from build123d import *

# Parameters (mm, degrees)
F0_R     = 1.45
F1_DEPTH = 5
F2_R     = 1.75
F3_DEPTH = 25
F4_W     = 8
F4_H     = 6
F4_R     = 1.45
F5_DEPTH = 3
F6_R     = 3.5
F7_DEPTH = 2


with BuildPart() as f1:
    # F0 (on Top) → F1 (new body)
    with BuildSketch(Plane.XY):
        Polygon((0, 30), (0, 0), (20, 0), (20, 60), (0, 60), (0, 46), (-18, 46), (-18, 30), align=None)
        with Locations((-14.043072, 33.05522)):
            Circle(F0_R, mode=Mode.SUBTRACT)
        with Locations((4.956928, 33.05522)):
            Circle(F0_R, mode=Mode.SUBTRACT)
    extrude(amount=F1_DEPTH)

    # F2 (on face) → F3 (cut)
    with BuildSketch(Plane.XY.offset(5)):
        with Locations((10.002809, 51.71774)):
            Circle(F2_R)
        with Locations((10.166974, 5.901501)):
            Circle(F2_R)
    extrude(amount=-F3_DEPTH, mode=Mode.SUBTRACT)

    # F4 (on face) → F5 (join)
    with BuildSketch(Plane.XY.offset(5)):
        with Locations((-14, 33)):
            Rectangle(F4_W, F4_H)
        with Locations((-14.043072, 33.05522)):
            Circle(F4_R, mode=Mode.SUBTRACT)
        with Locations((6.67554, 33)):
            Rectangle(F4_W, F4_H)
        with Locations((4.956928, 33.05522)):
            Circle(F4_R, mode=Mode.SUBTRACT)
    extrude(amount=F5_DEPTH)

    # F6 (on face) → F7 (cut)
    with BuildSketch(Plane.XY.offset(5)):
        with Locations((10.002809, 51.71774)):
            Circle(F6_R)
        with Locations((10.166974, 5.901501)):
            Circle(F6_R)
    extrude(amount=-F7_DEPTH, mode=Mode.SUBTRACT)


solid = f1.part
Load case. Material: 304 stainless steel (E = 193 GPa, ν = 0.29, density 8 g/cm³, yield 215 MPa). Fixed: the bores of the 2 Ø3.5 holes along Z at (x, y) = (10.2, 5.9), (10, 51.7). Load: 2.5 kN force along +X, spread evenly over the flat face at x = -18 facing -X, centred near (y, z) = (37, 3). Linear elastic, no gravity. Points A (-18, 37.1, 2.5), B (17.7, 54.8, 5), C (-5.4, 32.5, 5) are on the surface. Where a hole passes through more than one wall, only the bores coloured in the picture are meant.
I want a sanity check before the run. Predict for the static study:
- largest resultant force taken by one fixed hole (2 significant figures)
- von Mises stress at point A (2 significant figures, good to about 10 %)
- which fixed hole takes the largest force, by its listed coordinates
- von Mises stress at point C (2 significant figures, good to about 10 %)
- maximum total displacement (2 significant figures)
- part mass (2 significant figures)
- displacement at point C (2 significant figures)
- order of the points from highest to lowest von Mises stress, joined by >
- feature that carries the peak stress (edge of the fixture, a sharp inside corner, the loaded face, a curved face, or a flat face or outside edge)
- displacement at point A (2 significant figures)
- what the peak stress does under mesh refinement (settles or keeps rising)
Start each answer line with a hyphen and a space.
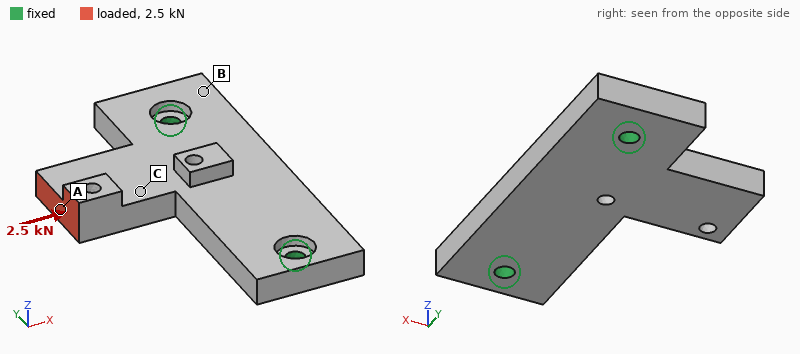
- 1.7 kN
- 39 MPa
- (10, 51.7)
- 71 MPa
- 45 µm
- 59 g
- 20 µm
- C > A > B
- edge of the fixture
- 38 µm
- keeps rising
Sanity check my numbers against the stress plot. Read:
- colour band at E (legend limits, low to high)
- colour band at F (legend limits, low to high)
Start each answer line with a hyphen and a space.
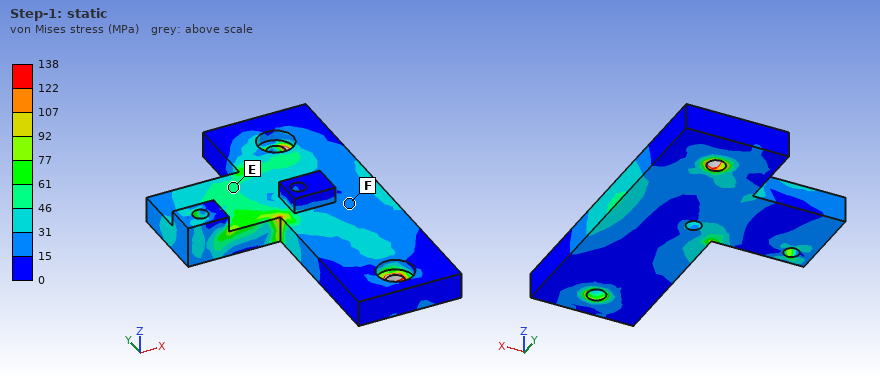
- 46 to 61 MPa
- 15 to 31 MPa
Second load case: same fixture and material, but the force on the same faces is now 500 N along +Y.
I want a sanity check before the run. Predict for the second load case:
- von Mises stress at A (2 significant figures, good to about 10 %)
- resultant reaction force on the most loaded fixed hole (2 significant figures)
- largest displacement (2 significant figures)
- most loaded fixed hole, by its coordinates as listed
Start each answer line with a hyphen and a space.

- 12 MPa
- 430 N
- 13 µm
- (10, 51.7)
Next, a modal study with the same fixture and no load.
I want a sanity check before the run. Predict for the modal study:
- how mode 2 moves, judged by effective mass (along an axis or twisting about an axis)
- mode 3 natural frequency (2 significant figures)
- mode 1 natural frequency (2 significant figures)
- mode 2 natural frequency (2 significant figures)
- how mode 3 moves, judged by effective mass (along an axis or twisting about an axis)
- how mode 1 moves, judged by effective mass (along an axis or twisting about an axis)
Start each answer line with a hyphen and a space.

- along Z
- 13 kHz
- 3700 Hz
- 8500 Hz
- along X
- along Z
